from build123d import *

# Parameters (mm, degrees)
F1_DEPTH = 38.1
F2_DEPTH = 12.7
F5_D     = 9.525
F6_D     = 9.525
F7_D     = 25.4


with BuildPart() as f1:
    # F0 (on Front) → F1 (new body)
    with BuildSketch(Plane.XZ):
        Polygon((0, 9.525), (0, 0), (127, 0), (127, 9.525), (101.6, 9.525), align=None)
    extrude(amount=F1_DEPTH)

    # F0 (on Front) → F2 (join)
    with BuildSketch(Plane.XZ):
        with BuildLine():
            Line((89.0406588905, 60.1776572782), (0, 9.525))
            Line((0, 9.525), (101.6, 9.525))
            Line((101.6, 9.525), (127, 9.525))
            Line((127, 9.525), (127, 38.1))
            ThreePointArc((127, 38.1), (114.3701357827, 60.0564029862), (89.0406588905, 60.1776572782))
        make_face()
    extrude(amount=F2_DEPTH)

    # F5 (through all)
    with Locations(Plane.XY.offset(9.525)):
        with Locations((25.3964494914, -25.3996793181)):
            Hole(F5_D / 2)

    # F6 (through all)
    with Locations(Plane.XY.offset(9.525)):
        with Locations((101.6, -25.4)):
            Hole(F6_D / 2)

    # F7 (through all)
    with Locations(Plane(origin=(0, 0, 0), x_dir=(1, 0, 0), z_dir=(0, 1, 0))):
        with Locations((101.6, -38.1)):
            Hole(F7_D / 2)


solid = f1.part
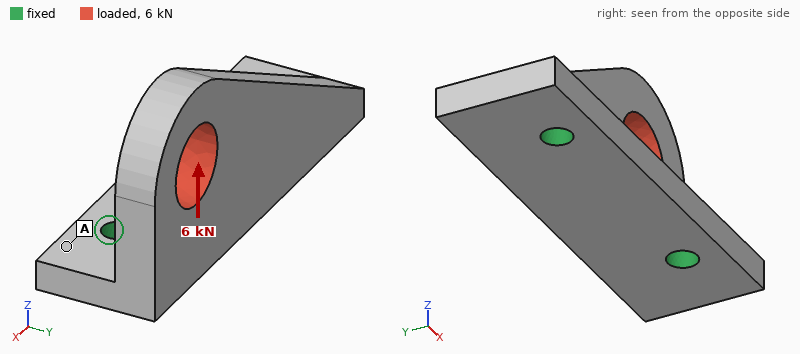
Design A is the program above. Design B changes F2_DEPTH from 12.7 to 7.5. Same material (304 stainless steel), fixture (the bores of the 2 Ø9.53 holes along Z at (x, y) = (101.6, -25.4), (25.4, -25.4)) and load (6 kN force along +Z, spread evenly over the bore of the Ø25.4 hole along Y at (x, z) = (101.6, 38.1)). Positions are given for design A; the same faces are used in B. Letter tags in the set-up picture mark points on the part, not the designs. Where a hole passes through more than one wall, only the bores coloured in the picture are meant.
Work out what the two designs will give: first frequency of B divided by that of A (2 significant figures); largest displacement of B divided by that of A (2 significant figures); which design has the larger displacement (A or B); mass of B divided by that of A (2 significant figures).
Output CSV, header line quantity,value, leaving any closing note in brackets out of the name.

quantity,value
first frequency of B divided by that of A,0.93
largest displacement of B divided by that of A,1.4
which design has the larger displacement,B
mass of B divided by that of A,0.79
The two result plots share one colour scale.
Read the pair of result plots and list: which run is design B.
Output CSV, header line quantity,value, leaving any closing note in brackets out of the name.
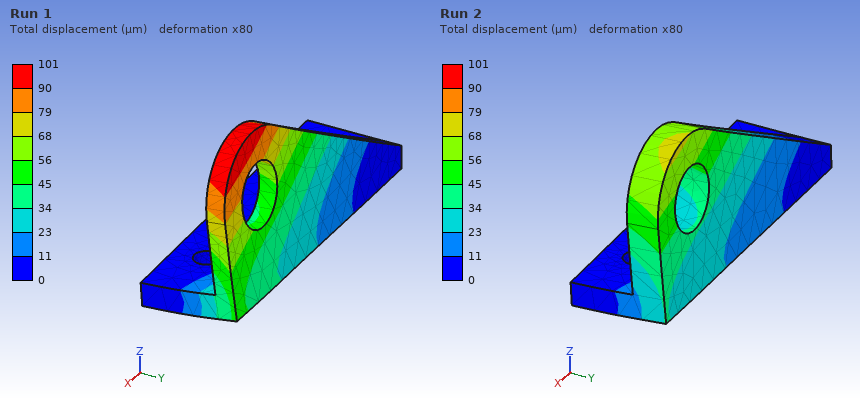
quantity,value
which run is design B,Run 1
